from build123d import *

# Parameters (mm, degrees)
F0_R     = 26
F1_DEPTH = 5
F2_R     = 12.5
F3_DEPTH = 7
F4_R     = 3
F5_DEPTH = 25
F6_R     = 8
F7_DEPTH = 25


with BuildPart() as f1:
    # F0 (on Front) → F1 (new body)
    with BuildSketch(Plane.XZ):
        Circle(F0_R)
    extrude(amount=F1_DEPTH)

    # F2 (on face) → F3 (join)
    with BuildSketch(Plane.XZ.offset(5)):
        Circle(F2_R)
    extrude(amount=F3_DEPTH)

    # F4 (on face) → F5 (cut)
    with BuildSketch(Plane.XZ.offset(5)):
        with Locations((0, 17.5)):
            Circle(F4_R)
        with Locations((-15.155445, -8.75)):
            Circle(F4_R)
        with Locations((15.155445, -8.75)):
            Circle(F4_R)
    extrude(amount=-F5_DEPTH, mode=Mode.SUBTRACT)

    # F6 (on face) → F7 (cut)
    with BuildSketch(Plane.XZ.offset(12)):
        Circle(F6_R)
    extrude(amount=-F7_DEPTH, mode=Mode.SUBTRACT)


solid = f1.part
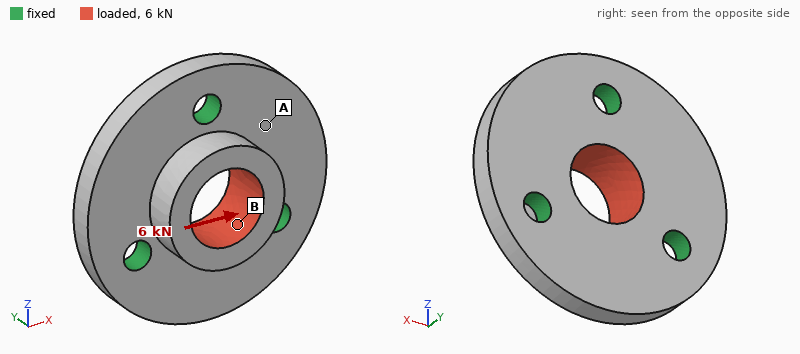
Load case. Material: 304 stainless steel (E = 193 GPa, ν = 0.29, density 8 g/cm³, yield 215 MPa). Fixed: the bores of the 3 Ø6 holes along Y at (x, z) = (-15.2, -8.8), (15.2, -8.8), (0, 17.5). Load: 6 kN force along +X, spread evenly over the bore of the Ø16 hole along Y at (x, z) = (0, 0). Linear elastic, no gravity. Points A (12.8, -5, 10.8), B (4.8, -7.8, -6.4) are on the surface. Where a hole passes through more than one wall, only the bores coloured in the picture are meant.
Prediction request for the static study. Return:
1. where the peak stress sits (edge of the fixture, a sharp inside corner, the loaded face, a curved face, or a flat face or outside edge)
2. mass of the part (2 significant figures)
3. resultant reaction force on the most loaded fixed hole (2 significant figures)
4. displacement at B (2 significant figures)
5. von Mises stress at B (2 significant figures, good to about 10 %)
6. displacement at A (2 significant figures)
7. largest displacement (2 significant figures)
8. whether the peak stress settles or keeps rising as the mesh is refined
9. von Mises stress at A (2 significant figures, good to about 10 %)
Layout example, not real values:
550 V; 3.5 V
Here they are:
edge of the fixture; 90 g; 2.1 kN; 2.1 µm; 34 MPa; 2.3 µm; 5.0 µm; keeps rising; 11 MPa
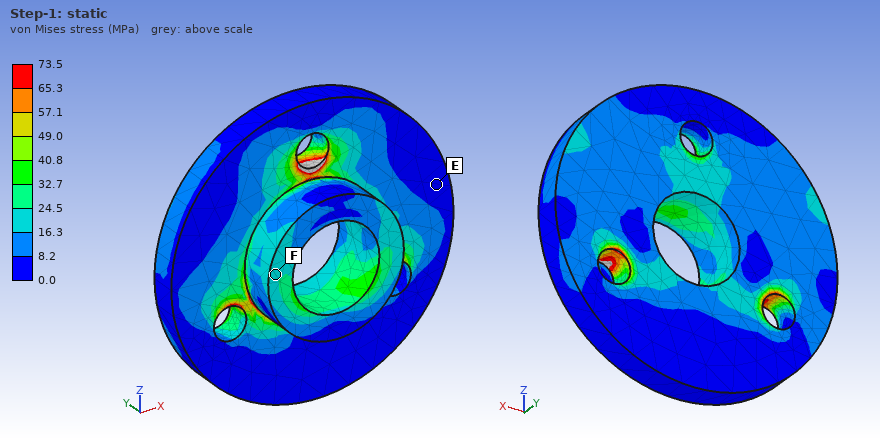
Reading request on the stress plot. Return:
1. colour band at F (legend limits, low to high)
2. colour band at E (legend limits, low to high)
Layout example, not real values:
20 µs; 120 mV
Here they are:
16.3 to 24.5 MPa; 0.0 to 8.2 MPa
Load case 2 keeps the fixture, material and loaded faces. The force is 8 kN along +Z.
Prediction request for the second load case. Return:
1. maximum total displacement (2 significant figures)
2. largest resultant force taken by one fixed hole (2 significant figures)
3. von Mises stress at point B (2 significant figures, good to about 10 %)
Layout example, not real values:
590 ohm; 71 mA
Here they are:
7.4 µm; 2.8 kN; 28 MPa
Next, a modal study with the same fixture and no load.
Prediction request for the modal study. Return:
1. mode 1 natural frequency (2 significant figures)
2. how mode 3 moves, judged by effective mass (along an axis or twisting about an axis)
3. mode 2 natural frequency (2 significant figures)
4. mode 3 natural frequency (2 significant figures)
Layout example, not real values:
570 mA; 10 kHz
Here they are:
15 kHz; along Y; 15 kHz; 17 kHz
